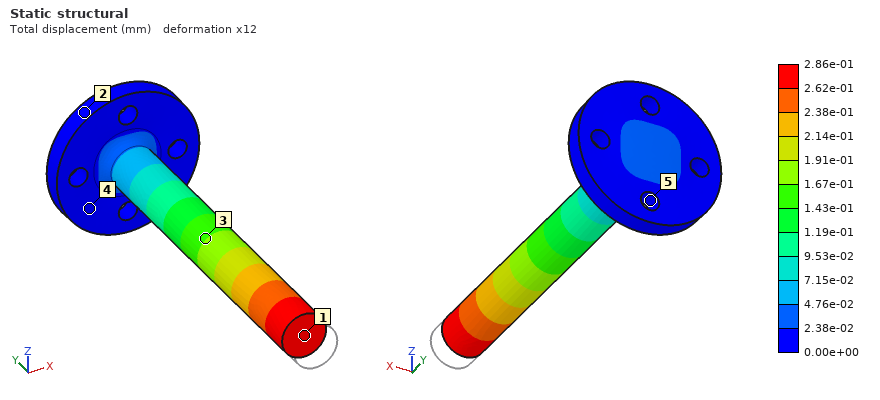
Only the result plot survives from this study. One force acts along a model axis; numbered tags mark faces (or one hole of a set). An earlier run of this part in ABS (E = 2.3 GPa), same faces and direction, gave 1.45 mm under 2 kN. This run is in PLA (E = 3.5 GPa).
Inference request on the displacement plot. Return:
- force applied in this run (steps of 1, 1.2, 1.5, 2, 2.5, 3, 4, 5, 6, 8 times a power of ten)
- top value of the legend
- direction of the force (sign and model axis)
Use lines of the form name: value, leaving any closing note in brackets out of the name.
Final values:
force applied in this run: 600 N
top value of the legend: 2.86e-01 mm
direction of the force: +Y
